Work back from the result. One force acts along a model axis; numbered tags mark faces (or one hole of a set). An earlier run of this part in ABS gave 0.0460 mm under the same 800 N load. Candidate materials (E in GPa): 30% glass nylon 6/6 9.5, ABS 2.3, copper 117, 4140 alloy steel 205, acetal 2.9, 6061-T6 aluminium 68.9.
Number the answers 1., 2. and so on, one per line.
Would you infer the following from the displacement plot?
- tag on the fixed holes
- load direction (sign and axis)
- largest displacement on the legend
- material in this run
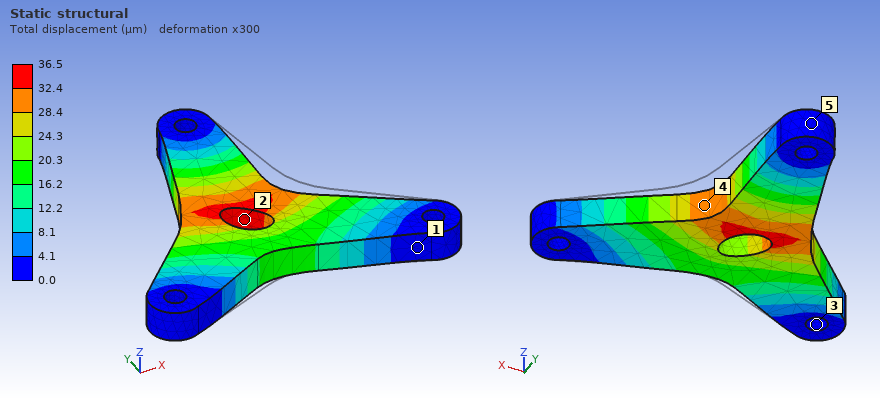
1. 3
2. -X
3. 36.5 µm
4. acetal
